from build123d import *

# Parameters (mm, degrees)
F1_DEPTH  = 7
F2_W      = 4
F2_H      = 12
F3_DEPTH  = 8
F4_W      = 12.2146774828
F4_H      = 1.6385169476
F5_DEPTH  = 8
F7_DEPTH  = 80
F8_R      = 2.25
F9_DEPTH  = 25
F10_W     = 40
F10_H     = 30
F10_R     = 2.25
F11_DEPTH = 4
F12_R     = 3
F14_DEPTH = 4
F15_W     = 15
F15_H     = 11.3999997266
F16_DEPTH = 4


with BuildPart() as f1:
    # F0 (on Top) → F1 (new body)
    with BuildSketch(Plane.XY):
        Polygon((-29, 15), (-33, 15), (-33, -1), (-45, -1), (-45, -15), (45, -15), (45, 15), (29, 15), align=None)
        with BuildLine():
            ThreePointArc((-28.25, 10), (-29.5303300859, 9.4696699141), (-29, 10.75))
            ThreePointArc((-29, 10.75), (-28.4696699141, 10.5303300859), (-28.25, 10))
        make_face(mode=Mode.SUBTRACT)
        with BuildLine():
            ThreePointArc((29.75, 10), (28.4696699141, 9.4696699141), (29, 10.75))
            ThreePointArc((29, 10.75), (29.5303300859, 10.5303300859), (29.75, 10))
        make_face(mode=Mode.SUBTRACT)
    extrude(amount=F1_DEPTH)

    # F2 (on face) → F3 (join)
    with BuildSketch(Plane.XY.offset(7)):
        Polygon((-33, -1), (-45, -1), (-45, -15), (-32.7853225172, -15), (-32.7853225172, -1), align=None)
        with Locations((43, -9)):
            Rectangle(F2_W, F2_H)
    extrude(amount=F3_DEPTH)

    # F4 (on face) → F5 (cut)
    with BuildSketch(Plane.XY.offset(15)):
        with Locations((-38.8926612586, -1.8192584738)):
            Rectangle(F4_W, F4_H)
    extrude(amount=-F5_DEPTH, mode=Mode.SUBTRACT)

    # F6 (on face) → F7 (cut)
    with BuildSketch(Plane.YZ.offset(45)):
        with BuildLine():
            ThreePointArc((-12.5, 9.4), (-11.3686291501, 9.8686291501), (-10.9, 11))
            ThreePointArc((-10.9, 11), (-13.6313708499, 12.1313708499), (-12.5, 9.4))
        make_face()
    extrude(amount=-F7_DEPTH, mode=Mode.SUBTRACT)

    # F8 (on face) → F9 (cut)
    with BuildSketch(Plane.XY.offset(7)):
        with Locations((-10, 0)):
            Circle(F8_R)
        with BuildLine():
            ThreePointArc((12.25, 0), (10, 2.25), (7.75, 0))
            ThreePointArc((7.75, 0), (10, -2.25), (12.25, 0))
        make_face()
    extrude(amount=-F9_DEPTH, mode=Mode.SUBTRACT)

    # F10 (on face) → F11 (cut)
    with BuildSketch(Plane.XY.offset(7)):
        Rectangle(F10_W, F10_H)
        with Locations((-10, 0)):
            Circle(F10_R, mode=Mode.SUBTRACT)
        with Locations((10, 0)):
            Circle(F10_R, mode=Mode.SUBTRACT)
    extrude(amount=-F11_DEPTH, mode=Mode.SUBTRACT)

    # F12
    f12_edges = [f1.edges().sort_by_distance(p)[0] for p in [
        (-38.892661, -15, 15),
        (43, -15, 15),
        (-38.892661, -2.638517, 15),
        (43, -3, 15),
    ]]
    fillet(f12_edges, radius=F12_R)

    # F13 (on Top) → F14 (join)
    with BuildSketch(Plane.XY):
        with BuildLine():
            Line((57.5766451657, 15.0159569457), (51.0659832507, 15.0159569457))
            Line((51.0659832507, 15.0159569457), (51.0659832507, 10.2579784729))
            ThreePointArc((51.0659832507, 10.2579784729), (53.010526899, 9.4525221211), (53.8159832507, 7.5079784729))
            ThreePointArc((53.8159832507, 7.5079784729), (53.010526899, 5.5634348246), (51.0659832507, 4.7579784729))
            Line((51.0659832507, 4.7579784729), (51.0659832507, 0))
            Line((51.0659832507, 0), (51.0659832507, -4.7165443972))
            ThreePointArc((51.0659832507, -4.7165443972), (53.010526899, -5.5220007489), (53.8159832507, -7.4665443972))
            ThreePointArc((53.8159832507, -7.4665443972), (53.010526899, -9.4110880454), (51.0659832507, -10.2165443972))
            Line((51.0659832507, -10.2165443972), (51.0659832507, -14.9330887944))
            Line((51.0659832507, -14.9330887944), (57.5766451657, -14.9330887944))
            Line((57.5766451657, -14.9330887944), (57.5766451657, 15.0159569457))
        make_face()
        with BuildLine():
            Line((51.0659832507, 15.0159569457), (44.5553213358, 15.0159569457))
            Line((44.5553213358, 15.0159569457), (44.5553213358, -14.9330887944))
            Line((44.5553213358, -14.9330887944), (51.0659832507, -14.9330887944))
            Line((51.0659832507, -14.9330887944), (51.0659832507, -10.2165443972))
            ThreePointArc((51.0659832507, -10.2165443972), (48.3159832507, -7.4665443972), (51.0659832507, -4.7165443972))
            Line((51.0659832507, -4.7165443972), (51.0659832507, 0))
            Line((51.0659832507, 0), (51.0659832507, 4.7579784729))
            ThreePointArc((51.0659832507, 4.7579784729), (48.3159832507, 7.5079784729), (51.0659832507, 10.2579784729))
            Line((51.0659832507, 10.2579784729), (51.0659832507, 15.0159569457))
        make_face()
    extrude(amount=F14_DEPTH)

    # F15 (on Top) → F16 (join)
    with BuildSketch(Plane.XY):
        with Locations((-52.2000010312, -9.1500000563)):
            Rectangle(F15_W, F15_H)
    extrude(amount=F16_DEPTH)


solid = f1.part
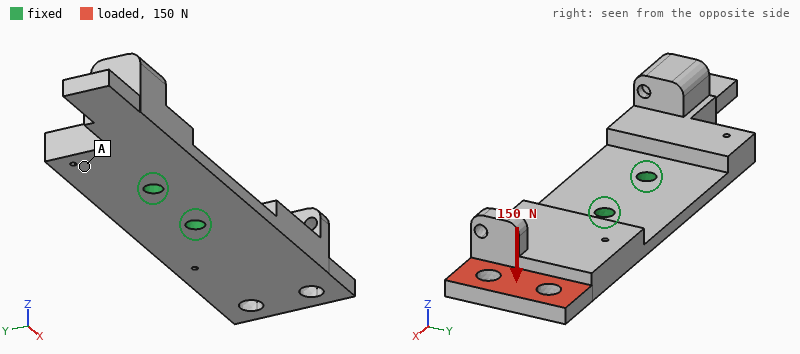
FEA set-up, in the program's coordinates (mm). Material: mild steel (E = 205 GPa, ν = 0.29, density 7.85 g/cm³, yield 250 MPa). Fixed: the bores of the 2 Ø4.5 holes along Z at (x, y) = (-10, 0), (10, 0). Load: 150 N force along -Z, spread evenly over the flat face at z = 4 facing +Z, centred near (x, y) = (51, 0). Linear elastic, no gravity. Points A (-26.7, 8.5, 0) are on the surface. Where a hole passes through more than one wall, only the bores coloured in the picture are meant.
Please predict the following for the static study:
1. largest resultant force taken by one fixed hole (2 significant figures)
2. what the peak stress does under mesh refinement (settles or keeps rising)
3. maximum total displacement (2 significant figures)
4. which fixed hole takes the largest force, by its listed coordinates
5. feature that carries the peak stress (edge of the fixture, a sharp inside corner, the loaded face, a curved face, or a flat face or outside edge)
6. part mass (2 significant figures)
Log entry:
240 N
keeps rising
0.20 mm
(10, 0)
edge of the fixture
130 g
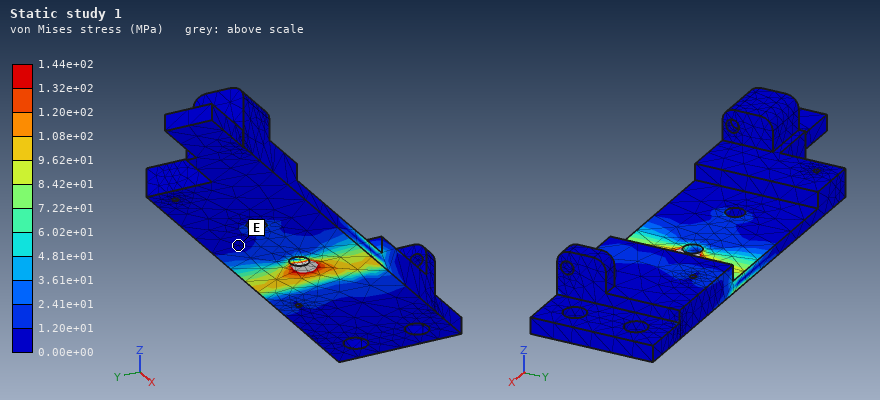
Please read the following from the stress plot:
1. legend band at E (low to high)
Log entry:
0.00e+00 to 1.20e+01 MPa
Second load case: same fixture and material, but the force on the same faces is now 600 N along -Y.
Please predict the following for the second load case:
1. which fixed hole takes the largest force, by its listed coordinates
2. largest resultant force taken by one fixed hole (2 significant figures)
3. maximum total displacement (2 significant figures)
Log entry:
(10, 0)
1.5 kN
31 µm
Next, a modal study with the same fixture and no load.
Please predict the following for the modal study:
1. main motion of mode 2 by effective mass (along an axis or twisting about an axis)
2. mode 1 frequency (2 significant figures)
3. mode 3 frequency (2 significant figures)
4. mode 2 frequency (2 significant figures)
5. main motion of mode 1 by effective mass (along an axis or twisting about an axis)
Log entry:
along Z
990 Hz
3400 Hz
1100 Hz
along Z
